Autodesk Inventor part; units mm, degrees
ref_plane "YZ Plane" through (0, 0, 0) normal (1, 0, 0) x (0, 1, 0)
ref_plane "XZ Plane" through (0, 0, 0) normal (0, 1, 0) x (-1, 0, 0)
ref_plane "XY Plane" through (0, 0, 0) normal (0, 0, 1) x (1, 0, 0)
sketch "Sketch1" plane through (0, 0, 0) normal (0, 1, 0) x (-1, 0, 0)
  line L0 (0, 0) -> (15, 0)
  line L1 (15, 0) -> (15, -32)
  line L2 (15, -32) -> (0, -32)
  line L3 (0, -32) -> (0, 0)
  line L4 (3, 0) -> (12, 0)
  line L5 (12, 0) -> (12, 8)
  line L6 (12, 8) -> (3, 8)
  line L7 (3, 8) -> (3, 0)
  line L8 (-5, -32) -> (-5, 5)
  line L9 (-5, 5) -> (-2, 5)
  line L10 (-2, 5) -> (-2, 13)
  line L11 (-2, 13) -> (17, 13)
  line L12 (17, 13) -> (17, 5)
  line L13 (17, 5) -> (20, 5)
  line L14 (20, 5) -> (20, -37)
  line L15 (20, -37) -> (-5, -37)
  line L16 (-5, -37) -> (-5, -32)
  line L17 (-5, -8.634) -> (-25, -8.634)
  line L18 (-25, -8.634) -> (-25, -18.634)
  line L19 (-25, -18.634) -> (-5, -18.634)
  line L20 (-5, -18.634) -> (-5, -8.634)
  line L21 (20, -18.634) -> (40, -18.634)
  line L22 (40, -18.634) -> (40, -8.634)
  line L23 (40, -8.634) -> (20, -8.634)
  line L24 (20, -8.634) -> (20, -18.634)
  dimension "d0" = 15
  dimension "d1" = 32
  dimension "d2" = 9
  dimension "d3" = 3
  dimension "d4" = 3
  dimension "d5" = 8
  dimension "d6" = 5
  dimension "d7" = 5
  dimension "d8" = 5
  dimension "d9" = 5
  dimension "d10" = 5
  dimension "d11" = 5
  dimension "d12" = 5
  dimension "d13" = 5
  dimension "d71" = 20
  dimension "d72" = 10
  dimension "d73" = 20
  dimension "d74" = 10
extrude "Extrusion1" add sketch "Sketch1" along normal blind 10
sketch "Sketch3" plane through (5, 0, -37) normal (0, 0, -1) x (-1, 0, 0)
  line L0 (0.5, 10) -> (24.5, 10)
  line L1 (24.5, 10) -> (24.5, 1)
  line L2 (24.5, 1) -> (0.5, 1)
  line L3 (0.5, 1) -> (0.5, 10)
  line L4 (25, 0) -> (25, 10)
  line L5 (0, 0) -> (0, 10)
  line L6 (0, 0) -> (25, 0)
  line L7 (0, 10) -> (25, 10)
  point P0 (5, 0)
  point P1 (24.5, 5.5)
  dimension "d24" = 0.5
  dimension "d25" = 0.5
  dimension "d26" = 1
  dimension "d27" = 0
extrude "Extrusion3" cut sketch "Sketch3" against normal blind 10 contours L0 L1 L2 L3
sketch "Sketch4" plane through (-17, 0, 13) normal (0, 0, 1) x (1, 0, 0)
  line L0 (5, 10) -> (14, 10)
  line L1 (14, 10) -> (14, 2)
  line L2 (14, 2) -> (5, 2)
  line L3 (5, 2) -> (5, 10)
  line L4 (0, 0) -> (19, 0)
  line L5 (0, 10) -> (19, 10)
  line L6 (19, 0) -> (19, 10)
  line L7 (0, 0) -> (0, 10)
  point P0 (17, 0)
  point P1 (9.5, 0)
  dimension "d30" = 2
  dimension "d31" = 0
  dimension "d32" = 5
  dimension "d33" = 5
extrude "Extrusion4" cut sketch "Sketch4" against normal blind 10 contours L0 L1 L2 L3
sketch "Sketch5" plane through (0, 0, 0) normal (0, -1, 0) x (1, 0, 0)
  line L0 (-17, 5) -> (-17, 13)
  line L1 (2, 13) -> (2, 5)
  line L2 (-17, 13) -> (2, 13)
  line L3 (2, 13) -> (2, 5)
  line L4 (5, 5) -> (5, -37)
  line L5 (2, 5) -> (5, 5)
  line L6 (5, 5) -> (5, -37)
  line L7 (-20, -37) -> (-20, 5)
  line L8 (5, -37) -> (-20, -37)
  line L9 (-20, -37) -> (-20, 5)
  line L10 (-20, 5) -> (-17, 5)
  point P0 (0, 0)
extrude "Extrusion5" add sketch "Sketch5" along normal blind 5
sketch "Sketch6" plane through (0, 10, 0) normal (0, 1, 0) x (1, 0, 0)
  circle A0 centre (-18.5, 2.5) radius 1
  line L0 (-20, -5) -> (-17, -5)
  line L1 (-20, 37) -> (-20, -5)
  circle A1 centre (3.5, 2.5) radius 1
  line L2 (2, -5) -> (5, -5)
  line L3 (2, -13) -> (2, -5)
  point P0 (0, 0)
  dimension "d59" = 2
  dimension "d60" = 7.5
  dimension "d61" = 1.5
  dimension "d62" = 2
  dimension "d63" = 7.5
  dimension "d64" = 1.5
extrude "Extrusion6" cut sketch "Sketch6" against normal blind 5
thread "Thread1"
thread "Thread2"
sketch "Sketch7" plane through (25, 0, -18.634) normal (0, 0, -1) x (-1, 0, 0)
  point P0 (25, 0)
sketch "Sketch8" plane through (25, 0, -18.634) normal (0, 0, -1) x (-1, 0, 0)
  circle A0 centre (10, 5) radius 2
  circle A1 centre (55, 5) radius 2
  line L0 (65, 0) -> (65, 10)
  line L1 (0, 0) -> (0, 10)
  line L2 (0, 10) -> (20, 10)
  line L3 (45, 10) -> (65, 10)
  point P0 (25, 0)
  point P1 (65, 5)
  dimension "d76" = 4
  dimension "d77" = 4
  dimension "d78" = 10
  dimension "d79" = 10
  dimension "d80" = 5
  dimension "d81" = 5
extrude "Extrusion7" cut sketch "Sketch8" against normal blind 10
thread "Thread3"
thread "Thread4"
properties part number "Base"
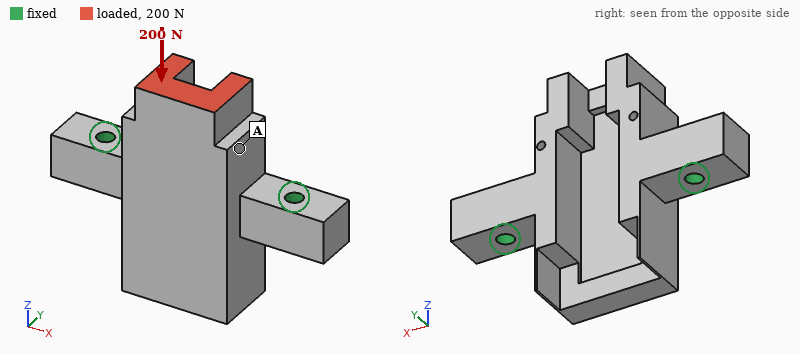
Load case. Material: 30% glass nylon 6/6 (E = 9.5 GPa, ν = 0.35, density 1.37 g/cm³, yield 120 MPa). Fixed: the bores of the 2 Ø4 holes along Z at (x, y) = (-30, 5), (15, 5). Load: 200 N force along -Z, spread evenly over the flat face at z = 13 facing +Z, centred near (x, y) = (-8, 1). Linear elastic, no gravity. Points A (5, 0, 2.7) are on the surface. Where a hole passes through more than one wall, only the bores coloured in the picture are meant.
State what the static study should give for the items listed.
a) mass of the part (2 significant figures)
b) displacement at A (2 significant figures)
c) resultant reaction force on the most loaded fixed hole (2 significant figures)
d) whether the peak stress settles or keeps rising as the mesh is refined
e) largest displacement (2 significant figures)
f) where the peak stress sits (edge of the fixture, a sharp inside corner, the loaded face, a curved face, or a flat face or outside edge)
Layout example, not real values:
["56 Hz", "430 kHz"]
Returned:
["20 g", "17 µm", "100 N", "keeps rising", "29 µm", "edge of the fixture"]
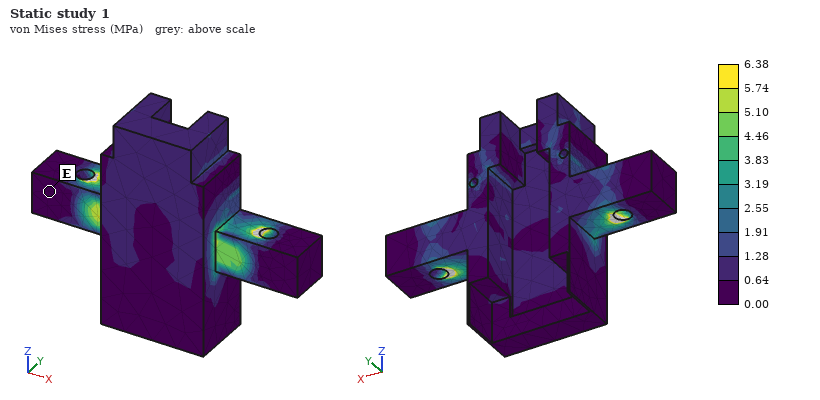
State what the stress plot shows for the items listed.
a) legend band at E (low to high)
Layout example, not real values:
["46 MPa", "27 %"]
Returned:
["0.00 to 0.64 MPa"]
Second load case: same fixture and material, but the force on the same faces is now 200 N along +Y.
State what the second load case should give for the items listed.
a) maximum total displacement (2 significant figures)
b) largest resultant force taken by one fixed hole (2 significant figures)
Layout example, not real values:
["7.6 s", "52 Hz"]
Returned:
["0.22 mm", "150 N"]
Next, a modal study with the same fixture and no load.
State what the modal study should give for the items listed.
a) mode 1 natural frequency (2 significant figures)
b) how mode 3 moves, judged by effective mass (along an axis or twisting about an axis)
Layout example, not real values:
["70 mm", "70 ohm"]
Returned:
["2500 Hz", "along Y"]
